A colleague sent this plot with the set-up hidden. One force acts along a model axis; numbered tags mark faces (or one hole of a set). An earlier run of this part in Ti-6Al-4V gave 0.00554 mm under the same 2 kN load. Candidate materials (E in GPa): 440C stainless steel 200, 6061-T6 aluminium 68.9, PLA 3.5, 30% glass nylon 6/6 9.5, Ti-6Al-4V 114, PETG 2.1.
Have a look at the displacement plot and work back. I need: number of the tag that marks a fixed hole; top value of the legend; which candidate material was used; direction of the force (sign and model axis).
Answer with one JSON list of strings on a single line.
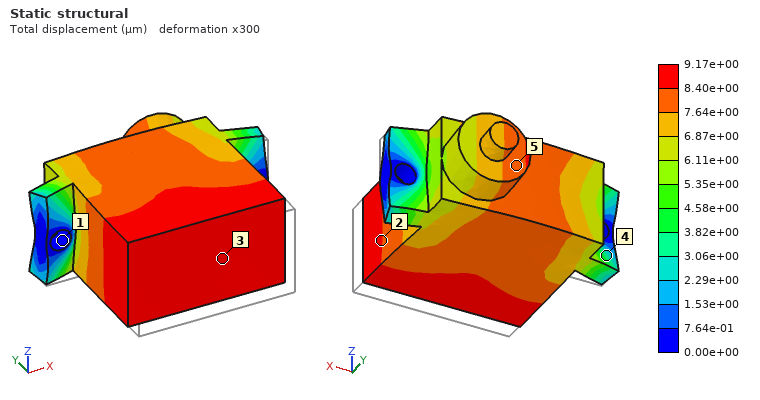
["1", "9.17e+00 µm", "6061-T6 aluminium", "+Y"]
